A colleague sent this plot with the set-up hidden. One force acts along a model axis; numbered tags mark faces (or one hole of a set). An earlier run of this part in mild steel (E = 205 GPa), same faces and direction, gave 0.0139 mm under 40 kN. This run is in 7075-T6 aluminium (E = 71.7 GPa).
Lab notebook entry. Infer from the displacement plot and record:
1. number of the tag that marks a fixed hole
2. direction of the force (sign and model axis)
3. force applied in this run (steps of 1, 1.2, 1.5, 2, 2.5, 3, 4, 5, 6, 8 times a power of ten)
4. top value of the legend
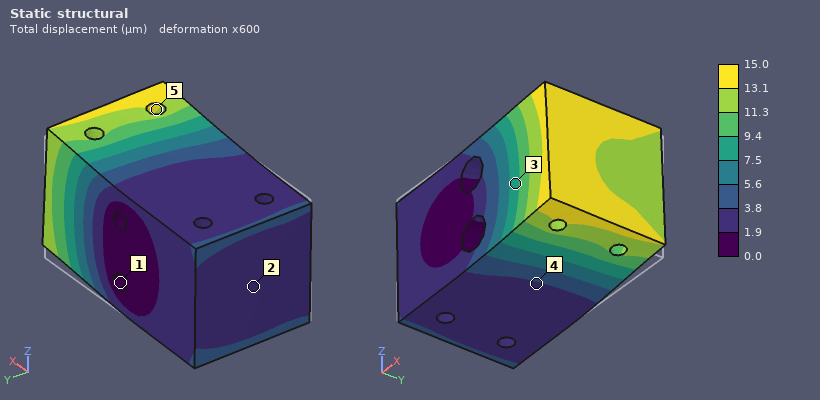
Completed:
1
+Z
15 kN
15.0 µm
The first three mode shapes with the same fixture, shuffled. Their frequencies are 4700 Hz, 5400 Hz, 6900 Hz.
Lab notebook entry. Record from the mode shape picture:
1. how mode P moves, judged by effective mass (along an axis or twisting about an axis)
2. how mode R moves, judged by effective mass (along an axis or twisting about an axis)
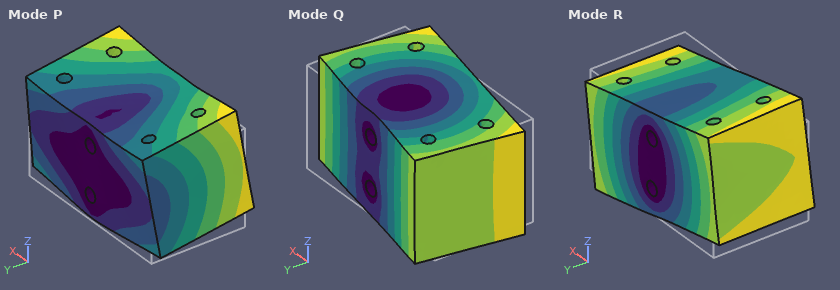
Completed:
along Z
twisting about Y
